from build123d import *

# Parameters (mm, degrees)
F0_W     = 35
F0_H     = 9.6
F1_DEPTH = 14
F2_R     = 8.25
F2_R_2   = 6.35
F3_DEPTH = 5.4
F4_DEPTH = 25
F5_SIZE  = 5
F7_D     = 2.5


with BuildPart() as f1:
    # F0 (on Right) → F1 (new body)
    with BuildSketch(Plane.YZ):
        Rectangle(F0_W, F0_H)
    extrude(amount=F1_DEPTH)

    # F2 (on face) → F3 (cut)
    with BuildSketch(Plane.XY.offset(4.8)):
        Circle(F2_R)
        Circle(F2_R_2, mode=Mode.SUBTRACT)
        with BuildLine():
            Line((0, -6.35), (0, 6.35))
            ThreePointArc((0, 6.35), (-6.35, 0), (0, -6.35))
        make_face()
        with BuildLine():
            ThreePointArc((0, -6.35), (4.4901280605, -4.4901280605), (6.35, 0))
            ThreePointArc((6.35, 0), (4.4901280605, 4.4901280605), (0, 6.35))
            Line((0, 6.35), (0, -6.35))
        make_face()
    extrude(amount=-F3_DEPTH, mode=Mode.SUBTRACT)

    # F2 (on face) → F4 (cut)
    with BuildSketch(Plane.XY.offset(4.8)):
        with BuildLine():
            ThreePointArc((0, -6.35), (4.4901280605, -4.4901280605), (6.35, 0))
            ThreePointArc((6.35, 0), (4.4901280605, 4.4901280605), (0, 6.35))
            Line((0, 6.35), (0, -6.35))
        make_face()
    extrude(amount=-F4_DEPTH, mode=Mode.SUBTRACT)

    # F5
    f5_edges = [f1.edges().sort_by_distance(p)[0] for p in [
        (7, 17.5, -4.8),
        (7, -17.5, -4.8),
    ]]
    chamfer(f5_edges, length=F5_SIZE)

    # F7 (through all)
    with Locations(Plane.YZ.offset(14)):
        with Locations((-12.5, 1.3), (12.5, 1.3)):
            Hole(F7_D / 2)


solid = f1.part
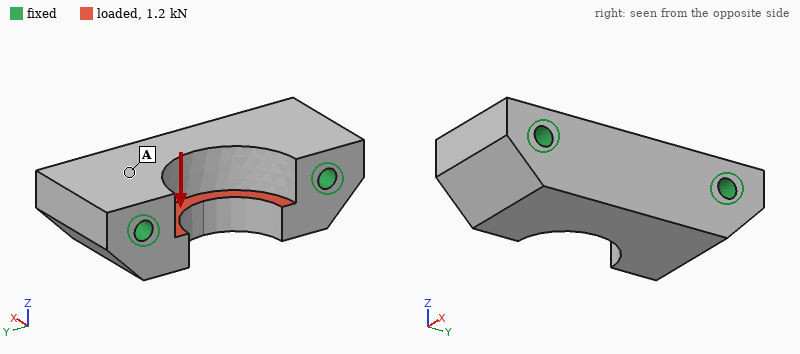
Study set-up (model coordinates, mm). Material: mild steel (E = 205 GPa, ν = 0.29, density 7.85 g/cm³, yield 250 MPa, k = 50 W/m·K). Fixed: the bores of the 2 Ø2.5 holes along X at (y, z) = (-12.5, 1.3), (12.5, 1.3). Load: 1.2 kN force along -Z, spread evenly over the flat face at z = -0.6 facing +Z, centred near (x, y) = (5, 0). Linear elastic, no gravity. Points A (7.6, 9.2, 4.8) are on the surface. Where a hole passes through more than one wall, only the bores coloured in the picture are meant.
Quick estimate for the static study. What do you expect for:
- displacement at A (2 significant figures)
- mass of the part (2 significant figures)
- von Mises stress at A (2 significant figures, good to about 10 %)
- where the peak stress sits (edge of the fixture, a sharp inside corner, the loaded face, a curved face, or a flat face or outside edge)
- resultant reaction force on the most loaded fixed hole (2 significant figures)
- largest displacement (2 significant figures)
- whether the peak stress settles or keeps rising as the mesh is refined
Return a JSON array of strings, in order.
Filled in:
["0.64 µm", "26 g", "8.0 MPa", "edge of the fixture", "640 N", "2.5 µm", "keeps rising"]
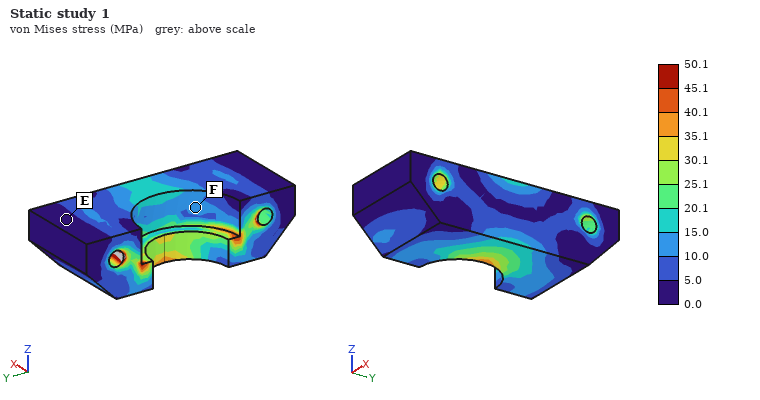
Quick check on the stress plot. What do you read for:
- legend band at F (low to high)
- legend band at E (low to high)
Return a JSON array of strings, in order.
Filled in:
["10.0 to 15.0 MPa", "0.0 to 5.0 MPa"]
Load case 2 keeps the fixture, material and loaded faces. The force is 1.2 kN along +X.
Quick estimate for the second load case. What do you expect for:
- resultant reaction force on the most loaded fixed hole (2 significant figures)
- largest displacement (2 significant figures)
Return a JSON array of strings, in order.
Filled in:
["610 N", "1.9 µm"]
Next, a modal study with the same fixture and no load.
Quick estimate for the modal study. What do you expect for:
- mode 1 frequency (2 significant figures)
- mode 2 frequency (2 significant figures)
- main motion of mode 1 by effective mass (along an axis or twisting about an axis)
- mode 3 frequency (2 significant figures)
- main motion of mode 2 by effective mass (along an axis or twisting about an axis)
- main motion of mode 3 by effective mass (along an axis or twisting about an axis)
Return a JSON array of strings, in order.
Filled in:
["42 kHz", "57 kHz", "along Z", "73 kHz", "along X", "twisting about Y"]
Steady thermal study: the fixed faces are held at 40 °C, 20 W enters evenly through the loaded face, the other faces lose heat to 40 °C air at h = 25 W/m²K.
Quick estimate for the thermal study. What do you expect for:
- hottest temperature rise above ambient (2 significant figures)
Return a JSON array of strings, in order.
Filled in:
["31 K"]
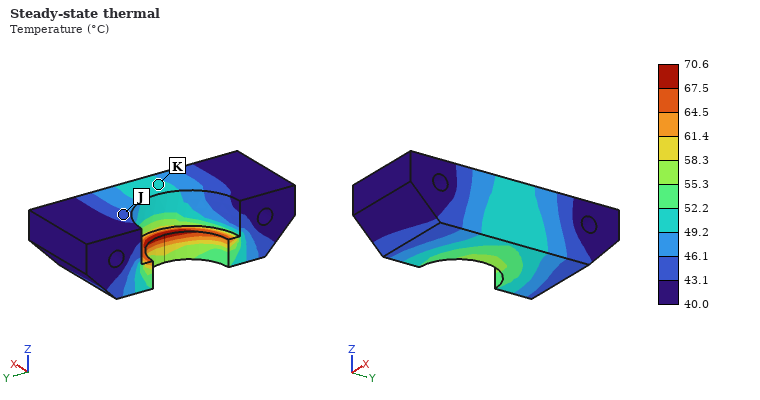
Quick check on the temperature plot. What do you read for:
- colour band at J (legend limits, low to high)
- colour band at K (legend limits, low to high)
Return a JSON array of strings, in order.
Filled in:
["43.1 to 46.1 °C", "49.2 to 52.2 °C"]
